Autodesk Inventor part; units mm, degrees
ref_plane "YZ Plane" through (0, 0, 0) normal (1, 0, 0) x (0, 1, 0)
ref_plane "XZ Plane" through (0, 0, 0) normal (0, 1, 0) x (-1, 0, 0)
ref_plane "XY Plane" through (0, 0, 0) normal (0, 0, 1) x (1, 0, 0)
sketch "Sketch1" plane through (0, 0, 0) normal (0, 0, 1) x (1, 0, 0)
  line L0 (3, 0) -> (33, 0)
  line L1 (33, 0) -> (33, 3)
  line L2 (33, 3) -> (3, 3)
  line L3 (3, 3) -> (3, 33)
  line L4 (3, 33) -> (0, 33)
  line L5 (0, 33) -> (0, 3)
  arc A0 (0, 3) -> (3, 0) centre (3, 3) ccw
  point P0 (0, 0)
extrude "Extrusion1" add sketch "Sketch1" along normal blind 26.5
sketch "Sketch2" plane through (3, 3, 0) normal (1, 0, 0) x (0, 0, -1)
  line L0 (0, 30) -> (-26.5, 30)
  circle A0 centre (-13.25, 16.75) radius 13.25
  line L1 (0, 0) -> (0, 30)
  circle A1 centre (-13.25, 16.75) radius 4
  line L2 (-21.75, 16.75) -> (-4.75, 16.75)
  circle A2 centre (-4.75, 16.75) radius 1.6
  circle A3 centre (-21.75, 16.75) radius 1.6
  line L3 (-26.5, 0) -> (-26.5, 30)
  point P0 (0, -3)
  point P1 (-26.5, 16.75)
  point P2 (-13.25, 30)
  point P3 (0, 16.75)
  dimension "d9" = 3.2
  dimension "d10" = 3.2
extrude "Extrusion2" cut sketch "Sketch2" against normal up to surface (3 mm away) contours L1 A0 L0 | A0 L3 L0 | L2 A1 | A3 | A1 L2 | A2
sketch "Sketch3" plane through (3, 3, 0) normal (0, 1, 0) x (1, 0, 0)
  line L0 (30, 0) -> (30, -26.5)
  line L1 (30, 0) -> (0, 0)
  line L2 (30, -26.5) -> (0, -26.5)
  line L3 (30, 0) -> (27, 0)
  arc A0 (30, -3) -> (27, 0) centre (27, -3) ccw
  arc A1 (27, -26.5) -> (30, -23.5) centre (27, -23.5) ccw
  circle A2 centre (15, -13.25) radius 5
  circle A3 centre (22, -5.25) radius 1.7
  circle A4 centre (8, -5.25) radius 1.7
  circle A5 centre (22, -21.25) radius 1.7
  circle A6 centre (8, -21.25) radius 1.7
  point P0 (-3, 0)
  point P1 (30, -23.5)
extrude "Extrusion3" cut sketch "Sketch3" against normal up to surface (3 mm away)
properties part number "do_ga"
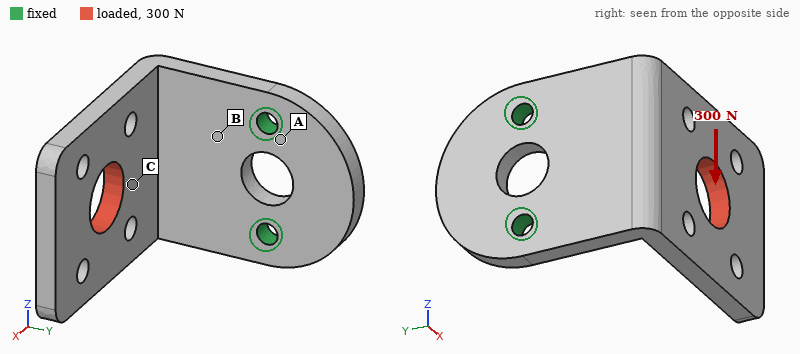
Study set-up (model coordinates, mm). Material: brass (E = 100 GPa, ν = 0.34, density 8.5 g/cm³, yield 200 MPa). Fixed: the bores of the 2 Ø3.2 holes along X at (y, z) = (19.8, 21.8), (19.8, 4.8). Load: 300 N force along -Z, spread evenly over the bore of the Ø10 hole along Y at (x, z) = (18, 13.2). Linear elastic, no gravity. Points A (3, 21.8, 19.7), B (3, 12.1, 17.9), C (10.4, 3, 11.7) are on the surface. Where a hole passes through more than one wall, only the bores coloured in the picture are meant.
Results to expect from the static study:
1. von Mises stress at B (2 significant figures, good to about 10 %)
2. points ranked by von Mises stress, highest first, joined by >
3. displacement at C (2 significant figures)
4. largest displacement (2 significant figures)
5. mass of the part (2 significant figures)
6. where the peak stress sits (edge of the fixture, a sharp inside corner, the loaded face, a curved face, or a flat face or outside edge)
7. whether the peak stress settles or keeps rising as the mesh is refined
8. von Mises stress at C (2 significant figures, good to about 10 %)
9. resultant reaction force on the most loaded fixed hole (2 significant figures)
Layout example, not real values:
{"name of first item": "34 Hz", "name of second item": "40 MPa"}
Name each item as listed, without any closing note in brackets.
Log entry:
{"von Mises stress at B": "74 MPa", "points ranked by von Mises stress, highest first, joined by >": "B > C > A", "displacement at C": "0.055 mm", "largest displacement": "0.19 mm", "mass of the part": "35 g", "where the peak stress sits": "edge of the fixture", "whether the peak stress settles or keeps rising as the mesh is refined": "keeps rising", "von Mises stress at C": "31 MPa", "resultant reaction force on the most loaded fixed hole": "400 N"}
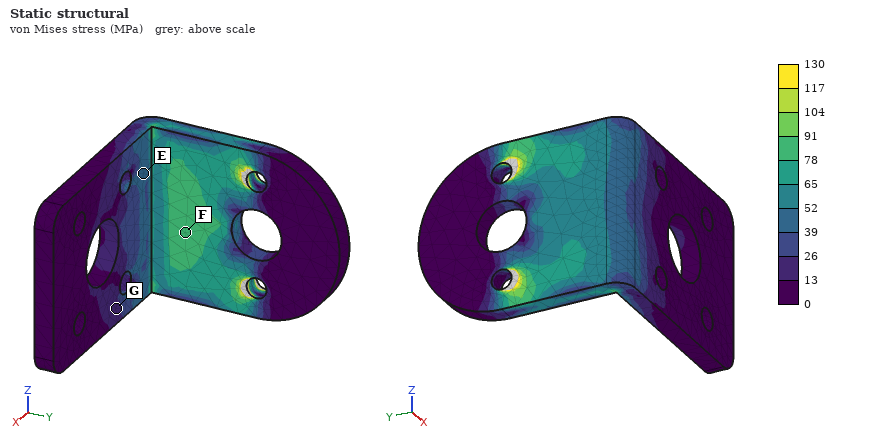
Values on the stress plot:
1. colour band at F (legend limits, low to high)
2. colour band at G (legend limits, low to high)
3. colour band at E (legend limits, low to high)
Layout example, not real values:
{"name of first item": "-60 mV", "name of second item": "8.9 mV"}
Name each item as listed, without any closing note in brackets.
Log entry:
{"colour band at F": "78 to 91 MPa", "colour band at G": "13 to 26 MPa", "colour band at E": "39 to 52 MPa"}
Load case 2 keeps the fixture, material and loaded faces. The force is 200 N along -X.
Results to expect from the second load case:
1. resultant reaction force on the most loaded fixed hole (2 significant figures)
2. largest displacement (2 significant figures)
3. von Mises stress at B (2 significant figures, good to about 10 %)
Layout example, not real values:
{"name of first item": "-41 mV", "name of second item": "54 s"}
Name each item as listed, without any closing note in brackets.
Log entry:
{"resultant reaction force on the most loaded fixed hole": "100 N", "largest displacement": "0.20 mm", "von Mises stress at B": "47 MPa"}
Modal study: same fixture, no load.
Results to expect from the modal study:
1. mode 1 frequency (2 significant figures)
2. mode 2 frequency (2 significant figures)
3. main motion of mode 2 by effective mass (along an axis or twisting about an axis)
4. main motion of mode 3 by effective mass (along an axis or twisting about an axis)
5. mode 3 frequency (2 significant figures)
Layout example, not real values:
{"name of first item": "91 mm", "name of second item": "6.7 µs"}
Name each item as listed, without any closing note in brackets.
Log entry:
{"mode 1 frequency": "900 Hz", "mode 2 frequency": "1700 Hz", "main motion of mode 2 by effective mass": "along Z", "main motion of mode 3 by effective mass": "along X", "mode 3 frequency": "2700 Hz"}
